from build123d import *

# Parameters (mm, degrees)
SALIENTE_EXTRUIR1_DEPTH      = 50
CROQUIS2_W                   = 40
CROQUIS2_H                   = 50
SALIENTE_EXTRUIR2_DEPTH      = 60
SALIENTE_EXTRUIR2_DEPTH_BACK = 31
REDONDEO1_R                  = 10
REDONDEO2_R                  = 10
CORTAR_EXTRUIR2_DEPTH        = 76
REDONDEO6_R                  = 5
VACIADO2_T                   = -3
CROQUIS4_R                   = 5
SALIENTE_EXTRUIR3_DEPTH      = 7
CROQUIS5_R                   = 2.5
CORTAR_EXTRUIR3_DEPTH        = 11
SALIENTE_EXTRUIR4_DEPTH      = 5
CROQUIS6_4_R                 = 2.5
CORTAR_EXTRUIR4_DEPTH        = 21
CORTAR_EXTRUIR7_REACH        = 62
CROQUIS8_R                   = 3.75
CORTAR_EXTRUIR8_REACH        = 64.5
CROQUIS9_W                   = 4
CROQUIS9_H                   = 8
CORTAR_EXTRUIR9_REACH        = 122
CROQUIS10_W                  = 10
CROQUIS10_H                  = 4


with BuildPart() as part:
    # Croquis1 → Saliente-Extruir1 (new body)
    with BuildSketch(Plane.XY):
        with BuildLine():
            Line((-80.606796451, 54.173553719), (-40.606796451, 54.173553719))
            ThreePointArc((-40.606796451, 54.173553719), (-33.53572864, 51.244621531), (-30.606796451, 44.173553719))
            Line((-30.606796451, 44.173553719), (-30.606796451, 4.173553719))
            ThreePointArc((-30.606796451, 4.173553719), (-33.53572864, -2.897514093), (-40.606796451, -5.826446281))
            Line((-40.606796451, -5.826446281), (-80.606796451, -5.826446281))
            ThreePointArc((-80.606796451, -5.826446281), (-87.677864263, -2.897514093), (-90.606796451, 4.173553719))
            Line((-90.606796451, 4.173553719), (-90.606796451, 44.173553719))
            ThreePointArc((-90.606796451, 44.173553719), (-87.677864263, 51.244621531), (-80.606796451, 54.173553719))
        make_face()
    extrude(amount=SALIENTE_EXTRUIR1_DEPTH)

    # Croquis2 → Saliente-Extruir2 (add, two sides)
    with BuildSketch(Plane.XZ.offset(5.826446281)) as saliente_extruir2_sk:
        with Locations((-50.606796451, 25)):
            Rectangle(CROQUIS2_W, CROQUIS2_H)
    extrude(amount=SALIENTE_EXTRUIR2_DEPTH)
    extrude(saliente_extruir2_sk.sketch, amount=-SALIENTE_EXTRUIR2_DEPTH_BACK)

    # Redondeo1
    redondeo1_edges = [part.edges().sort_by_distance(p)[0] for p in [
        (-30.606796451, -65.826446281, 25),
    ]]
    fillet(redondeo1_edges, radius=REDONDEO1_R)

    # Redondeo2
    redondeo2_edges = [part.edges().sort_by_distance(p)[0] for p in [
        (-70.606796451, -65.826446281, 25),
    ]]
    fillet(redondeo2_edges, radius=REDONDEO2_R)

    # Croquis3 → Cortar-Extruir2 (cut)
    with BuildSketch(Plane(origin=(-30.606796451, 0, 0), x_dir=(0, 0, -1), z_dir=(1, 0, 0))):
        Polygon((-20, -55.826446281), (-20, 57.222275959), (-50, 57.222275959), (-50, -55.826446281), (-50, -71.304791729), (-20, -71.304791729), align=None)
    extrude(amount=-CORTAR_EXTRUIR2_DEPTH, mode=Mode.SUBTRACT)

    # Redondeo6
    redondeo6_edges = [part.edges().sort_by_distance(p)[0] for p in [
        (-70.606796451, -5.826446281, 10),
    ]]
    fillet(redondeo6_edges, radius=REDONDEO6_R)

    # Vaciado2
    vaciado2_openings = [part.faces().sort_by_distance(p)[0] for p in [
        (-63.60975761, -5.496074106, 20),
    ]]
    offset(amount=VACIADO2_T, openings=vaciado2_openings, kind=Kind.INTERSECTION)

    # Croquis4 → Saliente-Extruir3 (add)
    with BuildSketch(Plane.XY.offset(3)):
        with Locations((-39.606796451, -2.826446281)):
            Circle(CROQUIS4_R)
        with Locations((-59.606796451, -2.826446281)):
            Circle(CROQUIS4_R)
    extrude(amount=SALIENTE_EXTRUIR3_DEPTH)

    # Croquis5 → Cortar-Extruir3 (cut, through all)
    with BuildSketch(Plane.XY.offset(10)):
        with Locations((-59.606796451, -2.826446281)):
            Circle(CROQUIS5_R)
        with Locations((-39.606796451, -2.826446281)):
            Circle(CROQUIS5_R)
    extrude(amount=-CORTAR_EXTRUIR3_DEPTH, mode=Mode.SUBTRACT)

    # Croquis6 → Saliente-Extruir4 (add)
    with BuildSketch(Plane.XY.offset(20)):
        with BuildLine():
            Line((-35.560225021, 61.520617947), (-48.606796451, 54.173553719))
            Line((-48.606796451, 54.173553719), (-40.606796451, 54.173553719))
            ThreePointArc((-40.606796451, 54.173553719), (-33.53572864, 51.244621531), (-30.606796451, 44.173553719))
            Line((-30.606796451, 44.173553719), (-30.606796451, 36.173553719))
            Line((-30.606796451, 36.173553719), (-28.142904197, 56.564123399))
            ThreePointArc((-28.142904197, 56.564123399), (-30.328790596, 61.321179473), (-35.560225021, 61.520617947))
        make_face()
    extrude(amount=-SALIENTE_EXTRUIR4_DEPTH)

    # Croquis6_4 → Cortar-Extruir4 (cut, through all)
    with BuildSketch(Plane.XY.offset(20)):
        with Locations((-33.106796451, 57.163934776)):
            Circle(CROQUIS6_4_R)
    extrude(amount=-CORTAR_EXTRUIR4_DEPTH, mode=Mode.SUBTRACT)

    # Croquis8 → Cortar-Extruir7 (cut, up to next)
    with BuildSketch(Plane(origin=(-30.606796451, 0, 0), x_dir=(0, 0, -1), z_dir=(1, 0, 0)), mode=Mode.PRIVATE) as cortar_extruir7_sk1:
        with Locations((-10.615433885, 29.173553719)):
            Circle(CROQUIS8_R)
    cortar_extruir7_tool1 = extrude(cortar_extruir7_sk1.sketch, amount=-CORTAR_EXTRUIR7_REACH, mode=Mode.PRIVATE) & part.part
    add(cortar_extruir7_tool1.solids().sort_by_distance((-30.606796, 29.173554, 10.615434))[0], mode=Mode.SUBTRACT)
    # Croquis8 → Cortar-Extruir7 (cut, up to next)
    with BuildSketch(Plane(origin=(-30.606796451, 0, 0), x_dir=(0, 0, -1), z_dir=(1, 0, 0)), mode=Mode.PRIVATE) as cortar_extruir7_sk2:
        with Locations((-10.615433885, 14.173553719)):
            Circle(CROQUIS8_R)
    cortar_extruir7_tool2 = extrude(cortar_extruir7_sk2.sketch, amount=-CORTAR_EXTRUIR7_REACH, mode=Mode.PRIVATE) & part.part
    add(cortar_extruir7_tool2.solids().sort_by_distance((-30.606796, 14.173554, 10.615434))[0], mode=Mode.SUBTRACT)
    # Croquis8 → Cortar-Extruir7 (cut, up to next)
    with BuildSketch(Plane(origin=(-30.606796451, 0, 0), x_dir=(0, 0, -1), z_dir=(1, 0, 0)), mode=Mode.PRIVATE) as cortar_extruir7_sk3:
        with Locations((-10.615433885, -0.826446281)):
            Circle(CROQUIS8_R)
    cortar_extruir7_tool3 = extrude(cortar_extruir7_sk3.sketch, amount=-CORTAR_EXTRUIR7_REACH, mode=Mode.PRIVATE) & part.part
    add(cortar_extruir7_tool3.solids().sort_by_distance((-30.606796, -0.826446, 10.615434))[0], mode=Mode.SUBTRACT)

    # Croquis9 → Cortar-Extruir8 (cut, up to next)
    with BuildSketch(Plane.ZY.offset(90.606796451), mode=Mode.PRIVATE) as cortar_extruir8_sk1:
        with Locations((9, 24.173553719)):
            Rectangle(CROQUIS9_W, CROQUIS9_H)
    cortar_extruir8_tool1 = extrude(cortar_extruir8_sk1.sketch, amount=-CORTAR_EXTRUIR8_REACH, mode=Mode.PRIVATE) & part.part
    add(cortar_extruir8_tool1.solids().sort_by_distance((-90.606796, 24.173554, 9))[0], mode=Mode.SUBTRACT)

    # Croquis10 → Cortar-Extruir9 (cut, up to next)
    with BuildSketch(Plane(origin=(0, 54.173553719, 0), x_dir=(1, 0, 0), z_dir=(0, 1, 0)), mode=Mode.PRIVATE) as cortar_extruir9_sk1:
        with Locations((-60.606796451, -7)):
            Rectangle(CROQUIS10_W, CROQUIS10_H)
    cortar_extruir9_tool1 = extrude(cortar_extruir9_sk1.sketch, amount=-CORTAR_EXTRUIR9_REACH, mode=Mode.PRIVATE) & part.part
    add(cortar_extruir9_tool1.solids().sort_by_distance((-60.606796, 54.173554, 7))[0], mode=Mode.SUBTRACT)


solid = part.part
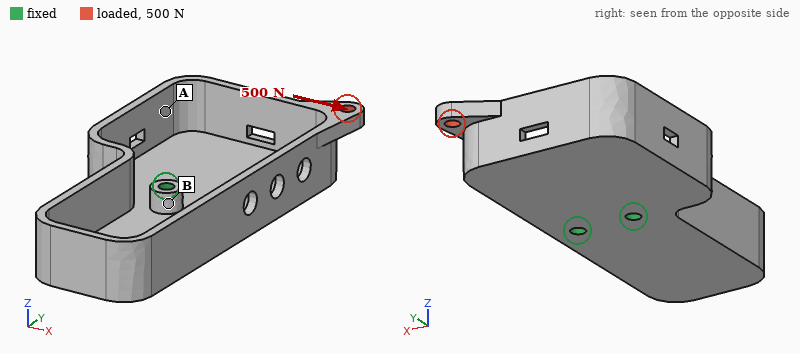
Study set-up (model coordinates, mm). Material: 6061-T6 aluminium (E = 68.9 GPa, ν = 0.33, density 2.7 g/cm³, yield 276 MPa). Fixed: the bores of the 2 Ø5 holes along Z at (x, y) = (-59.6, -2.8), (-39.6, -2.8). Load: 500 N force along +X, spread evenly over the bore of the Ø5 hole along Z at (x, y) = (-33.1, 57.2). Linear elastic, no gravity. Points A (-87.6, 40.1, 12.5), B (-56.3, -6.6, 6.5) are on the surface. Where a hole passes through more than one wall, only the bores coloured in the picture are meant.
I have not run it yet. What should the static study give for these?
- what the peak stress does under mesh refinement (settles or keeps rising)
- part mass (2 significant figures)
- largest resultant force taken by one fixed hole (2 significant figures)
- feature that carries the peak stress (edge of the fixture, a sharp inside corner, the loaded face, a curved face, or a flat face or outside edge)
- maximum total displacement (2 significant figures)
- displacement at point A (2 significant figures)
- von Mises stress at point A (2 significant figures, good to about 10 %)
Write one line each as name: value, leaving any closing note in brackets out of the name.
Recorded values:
what the peak stress does under mesh refinement: keeps rising
part mass: 95 g
largest resultant force taken by one fixed hole: 1.3 kN
feature that carries the peak stress: edge of the fixture
maximum total displacement: 0.36 mm
displacement at point A: 0.28 mm
von Mises stress at point A: 14 MPa
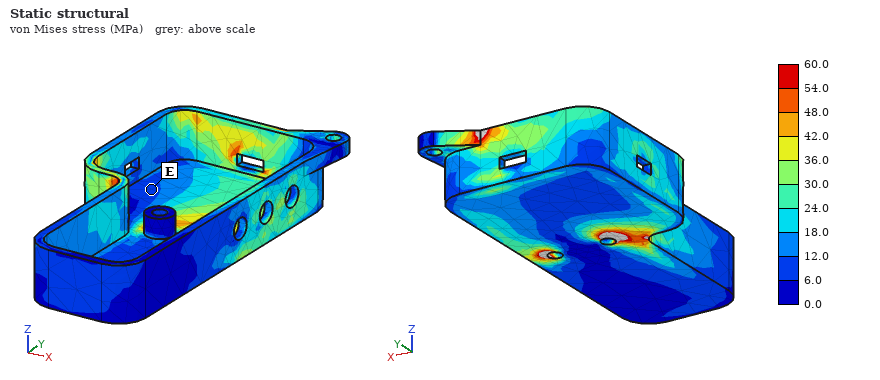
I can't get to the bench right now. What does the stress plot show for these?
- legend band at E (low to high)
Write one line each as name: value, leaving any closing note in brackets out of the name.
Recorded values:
legend band at E: 6.0 to 12.0 MPa
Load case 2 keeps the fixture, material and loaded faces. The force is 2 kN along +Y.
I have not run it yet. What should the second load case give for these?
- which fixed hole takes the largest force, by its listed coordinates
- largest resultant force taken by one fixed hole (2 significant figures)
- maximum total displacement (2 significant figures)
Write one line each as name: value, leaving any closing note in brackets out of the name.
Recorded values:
which fixed hole takes the largest force, by its listed coordinates: (-39.6, -2.8)
largest resultant force taken by one fixed hole: 2.4 kN
maximum total displacement: 0.96 mm
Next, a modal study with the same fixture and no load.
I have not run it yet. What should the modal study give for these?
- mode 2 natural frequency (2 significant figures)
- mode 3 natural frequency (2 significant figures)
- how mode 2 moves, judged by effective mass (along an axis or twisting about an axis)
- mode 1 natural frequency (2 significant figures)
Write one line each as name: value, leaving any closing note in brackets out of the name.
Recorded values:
mode 2 natural frequency: 1200 Hz
mode 3 natural frequency: 1500 Hz
how mode 2 moves, judged by effective mass: along Z
mode 1 natural frequency: 760 Hz
